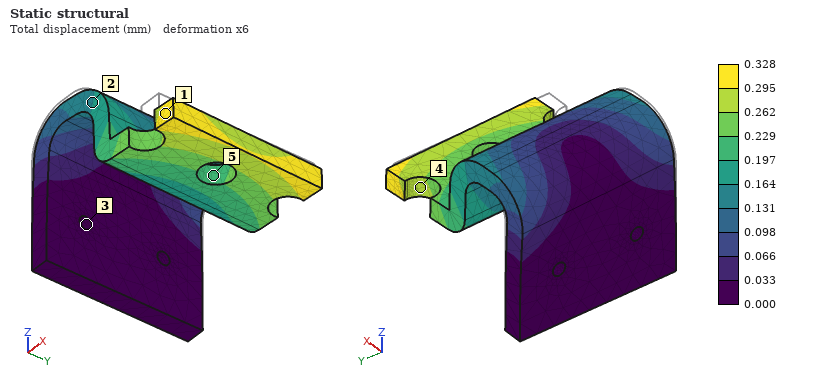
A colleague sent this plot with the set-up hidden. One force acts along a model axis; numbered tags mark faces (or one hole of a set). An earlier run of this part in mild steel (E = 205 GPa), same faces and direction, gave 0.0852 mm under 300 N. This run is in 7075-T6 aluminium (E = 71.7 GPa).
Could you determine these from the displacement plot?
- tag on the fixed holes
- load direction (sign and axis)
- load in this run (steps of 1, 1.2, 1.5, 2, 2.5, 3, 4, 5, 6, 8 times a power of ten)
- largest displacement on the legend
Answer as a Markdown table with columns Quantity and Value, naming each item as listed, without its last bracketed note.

| Quantity | Value |
|---|---|
| tag on the fixed holes | 3 |
| load direction | +Y |
| load in this run | 400 N |
| largest displacement on the legend | 0.328 mm |
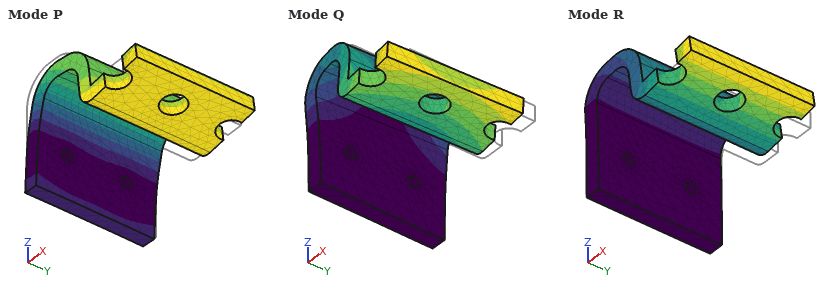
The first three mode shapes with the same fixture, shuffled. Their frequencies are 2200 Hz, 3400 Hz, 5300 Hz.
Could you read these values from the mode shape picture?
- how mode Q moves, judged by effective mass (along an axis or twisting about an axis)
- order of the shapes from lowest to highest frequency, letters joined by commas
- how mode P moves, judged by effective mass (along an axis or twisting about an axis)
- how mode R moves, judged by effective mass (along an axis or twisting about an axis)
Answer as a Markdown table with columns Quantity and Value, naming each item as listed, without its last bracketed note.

| Quantity | Value |
|---|---|
| how mode Q moves, judged by effective mass | along Y |
| order of the shapes from lowest to highest frequency, letters joined by commas | R, Q, P |
| how mode P moves, judged by effective mass | along X |
| how mode R moves, judged by effective mass | along Z |
